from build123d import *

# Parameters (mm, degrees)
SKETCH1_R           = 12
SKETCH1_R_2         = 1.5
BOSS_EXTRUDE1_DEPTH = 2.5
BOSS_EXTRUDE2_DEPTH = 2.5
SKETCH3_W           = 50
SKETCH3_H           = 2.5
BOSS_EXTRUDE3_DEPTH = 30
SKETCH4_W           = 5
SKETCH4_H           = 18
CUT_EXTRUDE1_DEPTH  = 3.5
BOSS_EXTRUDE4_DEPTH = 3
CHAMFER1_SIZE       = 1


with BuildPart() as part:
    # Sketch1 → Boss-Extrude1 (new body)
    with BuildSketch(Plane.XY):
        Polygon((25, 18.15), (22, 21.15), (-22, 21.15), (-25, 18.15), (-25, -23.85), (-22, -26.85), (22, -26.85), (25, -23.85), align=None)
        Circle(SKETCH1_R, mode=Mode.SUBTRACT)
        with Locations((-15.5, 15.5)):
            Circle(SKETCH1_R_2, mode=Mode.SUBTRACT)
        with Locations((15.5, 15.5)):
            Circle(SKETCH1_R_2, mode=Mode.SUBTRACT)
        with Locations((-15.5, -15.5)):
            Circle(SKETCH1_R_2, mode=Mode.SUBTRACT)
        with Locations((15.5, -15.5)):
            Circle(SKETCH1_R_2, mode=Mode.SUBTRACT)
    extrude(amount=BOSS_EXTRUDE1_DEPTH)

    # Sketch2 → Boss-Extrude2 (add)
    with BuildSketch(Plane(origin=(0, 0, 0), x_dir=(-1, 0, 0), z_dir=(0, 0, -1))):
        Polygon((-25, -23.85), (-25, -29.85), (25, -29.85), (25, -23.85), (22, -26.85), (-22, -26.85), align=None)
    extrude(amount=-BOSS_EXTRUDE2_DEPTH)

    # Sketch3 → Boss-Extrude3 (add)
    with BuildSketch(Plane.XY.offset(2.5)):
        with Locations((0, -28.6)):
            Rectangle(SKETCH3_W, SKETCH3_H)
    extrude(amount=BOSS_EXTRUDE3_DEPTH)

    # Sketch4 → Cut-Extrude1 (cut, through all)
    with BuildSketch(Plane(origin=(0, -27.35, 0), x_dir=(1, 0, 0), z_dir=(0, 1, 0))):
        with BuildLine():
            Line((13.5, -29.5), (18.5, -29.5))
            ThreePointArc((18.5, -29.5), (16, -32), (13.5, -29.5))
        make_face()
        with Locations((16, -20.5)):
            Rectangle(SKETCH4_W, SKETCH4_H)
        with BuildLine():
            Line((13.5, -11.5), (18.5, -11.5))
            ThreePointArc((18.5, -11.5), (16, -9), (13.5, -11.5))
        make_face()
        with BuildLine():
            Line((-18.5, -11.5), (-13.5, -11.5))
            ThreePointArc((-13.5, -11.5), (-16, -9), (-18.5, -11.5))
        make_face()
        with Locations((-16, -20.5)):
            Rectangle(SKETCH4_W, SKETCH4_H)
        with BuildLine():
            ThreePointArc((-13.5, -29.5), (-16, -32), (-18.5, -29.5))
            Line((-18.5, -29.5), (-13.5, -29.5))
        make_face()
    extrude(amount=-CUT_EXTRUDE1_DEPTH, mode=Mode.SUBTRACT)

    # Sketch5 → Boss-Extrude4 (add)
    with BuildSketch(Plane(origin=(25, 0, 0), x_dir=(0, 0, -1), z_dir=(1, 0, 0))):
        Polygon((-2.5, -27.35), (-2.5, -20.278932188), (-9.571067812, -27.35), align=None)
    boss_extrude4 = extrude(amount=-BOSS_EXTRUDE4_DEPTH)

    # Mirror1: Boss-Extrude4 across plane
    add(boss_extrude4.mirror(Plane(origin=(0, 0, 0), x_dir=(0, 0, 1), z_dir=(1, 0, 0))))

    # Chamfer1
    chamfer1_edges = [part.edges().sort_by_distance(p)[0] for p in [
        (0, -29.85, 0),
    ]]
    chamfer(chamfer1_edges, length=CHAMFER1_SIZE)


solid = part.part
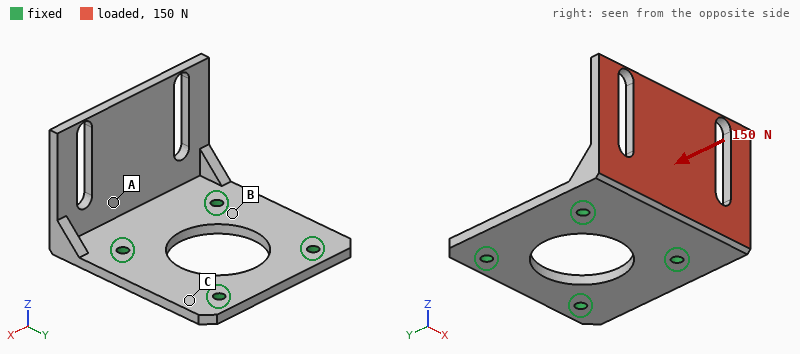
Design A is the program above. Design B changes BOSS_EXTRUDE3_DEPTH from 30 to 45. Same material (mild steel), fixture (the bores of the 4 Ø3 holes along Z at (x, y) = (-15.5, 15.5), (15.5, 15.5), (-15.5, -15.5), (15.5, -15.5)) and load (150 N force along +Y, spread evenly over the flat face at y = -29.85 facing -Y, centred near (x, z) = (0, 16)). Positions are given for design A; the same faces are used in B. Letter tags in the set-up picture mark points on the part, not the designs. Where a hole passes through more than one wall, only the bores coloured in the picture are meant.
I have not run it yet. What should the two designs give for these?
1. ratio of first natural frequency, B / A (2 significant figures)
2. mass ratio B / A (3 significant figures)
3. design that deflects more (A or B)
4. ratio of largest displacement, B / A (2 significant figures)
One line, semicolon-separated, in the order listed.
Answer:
0.48; 1.22; B; 2.8
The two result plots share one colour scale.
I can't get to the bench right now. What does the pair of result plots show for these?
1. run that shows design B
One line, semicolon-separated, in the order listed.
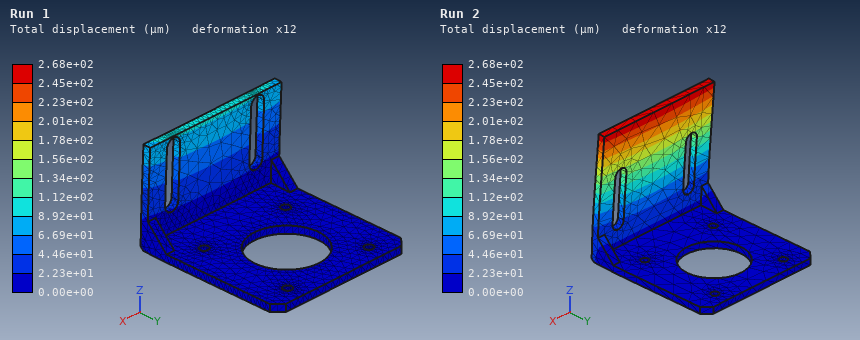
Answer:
Run 2
